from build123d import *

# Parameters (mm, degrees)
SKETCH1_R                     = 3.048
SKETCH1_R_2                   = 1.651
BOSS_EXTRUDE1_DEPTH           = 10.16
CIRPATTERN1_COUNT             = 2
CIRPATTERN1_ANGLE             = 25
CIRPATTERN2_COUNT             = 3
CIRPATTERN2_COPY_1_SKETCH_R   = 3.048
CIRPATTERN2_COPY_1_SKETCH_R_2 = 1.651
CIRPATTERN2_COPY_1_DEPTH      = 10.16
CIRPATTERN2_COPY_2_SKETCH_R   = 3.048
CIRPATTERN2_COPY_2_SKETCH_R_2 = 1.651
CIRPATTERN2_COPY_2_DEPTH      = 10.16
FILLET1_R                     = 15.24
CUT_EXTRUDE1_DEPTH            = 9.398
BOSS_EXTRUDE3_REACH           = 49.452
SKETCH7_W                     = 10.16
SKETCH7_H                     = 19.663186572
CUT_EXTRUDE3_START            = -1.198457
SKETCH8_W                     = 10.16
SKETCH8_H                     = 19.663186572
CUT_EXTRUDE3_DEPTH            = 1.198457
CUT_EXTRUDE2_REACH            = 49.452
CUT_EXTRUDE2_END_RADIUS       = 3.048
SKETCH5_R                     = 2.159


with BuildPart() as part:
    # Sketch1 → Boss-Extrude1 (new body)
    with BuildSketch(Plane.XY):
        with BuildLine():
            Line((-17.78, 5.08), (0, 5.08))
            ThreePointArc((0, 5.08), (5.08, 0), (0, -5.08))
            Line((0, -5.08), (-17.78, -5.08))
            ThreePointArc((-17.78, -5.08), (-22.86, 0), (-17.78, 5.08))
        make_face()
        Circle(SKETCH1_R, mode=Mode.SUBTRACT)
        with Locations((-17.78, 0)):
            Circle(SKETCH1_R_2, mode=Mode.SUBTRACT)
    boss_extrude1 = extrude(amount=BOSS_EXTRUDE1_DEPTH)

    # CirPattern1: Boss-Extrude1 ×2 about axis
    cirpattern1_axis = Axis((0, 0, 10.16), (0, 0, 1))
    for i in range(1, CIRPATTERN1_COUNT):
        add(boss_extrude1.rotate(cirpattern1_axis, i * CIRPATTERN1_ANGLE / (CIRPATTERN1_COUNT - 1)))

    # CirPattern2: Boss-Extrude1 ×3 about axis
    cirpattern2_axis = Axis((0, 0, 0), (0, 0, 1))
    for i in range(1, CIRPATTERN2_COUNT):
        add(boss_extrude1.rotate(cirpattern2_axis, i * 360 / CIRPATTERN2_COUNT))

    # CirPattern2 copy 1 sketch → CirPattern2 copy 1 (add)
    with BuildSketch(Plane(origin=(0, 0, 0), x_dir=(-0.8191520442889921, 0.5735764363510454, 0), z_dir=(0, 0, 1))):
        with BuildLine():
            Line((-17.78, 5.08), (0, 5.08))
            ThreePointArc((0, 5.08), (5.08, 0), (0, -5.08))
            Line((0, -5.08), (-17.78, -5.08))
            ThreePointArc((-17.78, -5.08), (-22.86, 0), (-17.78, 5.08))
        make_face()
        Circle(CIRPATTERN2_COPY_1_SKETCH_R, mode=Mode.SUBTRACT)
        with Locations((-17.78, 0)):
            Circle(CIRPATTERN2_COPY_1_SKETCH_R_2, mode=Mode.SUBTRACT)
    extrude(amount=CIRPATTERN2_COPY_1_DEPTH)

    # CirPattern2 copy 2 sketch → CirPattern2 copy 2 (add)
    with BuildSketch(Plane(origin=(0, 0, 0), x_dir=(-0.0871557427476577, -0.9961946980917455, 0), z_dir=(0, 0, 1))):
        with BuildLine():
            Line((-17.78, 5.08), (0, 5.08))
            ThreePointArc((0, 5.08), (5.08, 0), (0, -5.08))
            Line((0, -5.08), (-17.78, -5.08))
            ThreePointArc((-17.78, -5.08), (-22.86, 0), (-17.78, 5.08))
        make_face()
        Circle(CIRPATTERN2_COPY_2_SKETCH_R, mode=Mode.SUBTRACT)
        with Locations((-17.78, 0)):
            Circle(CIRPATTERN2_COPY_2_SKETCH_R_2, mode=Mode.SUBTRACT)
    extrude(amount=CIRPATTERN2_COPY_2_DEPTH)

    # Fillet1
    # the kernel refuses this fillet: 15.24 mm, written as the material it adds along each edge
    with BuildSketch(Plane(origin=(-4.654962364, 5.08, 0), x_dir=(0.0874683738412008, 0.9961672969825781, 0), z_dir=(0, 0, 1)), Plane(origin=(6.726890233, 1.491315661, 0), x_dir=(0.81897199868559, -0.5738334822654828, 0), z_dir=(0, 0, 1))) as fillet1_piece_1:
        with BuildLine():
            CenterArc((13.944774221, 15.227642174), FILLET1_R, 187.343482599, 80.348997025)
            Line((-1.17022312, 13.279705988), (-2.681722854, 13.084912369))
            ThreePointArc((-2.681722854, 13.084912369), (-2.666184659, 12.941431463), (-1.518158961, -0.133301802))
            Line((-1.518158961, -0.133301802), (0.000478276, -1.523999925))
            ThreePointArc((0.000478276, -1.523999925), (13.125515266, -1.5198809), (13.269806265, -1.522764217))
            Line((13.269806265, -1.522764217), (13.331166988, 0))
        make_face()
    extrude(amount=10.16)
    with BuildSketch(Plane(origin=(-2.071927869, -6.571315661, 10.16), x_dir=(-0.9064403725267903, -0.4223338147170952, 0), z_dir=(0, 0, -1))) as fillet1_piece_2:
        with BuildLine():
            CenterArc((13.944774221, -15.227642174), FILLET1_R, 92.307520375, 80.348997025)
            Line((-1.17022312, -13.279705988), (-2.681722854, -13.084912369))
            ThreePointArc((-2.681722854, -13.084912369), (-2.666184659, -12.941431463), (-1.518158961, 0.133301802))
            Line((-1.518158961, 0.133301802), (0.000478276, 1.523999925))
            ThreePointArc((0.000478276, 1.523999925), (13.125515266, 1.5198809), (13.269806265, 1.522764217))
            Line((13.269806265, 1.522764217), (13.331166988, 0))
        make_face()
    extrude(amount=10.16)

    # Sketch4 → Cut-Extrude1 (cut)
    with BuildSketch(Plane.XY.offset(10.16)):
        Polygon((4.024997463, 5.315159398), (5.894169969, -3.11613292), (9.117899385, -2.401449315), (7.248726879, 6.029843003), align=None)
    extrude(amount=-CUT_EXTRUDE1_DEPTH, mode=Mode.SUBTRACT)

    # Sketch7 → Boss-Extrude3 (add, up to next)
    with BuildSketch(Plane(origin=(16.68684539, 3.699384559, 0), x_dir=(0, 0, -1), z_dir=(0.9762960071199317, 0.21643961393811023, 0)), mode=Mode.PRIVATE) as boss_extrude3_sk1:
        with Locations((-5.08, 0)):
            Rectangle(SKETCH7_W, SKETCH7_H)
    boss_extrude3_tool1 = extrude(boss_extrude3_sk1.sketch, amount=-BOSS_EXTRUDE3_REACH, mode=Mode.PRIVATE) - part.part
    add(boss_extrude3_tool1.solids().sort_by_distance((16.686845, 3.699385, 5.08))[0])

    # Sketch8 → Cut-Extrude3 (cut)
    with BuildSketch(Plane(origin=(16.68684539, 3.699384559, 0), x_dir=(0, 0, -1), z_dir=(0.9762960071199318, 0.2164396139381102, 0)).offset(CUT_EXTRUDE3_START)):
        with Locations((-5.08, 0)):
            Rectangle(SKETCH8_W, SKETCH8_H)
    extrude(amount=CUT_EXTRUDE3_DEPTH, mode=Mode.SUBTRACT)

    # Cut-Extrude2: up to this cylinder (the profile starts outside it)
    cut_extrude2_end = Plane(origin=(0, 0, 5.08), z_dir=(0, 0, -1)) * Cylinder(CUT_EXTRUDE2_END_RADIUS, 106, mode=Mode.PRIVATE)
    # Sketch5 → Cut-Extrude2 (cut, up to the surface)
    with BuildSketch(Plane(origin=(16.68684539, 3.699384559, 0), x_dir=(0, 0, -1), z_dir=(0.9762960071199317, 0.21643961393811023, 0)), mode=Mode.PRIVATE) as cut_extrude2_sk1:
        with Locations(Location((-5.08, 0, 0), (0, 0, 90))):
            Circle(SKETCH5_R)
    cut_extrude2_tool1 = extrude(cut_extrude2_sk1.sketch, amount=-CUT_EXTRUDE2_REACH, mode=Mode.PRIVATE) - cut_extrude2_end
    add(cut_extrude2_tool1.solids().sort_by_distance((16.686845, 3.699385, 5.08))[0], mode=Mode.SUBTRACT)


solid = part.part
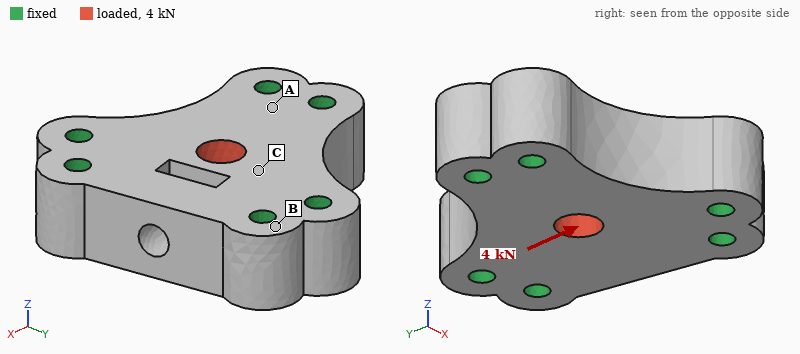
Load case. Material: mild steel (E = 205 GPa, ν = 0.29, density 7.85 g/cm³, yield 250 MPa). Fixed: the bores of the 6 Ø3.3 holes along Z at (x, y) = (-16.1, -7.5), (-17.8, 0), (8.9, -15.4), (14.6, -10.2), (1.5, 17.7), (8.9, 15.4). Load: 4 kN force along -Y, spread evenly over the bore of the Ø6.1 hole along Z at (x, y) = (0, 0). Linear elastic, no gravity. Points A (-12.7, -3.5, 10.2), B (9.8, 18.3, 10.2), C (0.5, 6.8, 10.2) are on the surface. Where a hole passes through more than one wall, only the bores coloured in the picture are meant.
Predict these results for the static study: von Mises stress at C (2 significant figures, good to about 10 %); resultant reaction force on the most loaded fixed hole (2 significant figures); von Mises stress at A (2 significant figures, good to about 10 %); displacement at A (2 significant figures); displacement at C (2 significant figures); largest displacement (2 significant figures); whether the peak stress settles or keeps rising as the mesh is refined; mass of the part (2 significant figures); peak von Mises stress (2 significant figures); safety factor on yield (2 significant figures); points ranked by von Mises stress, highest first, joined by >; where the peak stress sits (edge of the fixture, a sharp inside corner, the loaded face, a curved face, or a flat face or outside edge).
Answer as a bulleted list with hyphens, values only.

- 21 MPa
- 1.3 kN
- 12 MPa
- 0.29 µm
- 1.0 µm
- 1.9 µm
- settles
- 77 g
- 61 MPa
- 4.1
- C > A > B
- the loaded face
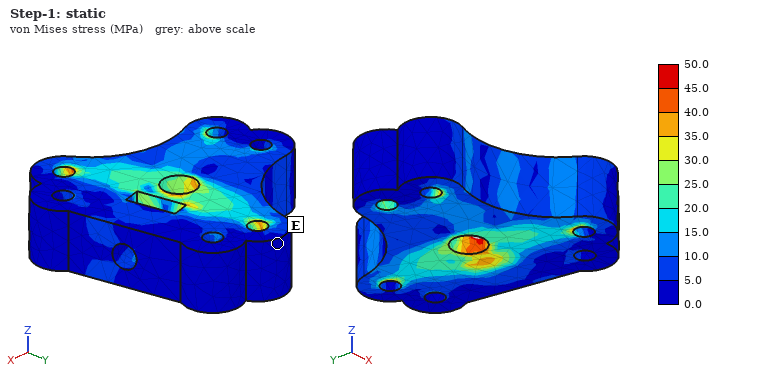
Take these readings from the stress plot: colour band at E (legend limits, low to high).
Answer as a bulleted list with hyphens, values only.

- 0.0 to 5.0 MPa
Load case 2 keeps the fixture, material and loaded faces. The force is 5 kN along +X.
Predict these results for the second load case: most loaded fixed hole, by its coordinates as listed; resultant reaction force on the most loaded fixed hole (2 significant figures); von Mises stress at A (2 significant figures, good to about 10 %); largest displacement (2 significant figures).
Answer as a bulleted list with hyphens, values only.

- (-17.8, 0)
- 1.5 kN
- 13 MPa
- 3.4 µm
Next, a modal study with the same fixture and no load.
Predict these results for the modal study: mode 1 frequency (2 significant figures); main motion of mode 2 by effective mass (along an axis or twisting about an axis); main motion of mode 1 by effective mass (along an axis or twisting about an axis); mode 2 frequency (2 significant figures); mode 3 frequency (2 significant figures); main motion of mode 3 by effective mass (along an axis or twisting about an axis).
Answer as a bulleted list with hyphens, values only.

- 41 kHz
- along Y
- along Z
- 53 kHz
- 56 kHz
- twisting about Y
